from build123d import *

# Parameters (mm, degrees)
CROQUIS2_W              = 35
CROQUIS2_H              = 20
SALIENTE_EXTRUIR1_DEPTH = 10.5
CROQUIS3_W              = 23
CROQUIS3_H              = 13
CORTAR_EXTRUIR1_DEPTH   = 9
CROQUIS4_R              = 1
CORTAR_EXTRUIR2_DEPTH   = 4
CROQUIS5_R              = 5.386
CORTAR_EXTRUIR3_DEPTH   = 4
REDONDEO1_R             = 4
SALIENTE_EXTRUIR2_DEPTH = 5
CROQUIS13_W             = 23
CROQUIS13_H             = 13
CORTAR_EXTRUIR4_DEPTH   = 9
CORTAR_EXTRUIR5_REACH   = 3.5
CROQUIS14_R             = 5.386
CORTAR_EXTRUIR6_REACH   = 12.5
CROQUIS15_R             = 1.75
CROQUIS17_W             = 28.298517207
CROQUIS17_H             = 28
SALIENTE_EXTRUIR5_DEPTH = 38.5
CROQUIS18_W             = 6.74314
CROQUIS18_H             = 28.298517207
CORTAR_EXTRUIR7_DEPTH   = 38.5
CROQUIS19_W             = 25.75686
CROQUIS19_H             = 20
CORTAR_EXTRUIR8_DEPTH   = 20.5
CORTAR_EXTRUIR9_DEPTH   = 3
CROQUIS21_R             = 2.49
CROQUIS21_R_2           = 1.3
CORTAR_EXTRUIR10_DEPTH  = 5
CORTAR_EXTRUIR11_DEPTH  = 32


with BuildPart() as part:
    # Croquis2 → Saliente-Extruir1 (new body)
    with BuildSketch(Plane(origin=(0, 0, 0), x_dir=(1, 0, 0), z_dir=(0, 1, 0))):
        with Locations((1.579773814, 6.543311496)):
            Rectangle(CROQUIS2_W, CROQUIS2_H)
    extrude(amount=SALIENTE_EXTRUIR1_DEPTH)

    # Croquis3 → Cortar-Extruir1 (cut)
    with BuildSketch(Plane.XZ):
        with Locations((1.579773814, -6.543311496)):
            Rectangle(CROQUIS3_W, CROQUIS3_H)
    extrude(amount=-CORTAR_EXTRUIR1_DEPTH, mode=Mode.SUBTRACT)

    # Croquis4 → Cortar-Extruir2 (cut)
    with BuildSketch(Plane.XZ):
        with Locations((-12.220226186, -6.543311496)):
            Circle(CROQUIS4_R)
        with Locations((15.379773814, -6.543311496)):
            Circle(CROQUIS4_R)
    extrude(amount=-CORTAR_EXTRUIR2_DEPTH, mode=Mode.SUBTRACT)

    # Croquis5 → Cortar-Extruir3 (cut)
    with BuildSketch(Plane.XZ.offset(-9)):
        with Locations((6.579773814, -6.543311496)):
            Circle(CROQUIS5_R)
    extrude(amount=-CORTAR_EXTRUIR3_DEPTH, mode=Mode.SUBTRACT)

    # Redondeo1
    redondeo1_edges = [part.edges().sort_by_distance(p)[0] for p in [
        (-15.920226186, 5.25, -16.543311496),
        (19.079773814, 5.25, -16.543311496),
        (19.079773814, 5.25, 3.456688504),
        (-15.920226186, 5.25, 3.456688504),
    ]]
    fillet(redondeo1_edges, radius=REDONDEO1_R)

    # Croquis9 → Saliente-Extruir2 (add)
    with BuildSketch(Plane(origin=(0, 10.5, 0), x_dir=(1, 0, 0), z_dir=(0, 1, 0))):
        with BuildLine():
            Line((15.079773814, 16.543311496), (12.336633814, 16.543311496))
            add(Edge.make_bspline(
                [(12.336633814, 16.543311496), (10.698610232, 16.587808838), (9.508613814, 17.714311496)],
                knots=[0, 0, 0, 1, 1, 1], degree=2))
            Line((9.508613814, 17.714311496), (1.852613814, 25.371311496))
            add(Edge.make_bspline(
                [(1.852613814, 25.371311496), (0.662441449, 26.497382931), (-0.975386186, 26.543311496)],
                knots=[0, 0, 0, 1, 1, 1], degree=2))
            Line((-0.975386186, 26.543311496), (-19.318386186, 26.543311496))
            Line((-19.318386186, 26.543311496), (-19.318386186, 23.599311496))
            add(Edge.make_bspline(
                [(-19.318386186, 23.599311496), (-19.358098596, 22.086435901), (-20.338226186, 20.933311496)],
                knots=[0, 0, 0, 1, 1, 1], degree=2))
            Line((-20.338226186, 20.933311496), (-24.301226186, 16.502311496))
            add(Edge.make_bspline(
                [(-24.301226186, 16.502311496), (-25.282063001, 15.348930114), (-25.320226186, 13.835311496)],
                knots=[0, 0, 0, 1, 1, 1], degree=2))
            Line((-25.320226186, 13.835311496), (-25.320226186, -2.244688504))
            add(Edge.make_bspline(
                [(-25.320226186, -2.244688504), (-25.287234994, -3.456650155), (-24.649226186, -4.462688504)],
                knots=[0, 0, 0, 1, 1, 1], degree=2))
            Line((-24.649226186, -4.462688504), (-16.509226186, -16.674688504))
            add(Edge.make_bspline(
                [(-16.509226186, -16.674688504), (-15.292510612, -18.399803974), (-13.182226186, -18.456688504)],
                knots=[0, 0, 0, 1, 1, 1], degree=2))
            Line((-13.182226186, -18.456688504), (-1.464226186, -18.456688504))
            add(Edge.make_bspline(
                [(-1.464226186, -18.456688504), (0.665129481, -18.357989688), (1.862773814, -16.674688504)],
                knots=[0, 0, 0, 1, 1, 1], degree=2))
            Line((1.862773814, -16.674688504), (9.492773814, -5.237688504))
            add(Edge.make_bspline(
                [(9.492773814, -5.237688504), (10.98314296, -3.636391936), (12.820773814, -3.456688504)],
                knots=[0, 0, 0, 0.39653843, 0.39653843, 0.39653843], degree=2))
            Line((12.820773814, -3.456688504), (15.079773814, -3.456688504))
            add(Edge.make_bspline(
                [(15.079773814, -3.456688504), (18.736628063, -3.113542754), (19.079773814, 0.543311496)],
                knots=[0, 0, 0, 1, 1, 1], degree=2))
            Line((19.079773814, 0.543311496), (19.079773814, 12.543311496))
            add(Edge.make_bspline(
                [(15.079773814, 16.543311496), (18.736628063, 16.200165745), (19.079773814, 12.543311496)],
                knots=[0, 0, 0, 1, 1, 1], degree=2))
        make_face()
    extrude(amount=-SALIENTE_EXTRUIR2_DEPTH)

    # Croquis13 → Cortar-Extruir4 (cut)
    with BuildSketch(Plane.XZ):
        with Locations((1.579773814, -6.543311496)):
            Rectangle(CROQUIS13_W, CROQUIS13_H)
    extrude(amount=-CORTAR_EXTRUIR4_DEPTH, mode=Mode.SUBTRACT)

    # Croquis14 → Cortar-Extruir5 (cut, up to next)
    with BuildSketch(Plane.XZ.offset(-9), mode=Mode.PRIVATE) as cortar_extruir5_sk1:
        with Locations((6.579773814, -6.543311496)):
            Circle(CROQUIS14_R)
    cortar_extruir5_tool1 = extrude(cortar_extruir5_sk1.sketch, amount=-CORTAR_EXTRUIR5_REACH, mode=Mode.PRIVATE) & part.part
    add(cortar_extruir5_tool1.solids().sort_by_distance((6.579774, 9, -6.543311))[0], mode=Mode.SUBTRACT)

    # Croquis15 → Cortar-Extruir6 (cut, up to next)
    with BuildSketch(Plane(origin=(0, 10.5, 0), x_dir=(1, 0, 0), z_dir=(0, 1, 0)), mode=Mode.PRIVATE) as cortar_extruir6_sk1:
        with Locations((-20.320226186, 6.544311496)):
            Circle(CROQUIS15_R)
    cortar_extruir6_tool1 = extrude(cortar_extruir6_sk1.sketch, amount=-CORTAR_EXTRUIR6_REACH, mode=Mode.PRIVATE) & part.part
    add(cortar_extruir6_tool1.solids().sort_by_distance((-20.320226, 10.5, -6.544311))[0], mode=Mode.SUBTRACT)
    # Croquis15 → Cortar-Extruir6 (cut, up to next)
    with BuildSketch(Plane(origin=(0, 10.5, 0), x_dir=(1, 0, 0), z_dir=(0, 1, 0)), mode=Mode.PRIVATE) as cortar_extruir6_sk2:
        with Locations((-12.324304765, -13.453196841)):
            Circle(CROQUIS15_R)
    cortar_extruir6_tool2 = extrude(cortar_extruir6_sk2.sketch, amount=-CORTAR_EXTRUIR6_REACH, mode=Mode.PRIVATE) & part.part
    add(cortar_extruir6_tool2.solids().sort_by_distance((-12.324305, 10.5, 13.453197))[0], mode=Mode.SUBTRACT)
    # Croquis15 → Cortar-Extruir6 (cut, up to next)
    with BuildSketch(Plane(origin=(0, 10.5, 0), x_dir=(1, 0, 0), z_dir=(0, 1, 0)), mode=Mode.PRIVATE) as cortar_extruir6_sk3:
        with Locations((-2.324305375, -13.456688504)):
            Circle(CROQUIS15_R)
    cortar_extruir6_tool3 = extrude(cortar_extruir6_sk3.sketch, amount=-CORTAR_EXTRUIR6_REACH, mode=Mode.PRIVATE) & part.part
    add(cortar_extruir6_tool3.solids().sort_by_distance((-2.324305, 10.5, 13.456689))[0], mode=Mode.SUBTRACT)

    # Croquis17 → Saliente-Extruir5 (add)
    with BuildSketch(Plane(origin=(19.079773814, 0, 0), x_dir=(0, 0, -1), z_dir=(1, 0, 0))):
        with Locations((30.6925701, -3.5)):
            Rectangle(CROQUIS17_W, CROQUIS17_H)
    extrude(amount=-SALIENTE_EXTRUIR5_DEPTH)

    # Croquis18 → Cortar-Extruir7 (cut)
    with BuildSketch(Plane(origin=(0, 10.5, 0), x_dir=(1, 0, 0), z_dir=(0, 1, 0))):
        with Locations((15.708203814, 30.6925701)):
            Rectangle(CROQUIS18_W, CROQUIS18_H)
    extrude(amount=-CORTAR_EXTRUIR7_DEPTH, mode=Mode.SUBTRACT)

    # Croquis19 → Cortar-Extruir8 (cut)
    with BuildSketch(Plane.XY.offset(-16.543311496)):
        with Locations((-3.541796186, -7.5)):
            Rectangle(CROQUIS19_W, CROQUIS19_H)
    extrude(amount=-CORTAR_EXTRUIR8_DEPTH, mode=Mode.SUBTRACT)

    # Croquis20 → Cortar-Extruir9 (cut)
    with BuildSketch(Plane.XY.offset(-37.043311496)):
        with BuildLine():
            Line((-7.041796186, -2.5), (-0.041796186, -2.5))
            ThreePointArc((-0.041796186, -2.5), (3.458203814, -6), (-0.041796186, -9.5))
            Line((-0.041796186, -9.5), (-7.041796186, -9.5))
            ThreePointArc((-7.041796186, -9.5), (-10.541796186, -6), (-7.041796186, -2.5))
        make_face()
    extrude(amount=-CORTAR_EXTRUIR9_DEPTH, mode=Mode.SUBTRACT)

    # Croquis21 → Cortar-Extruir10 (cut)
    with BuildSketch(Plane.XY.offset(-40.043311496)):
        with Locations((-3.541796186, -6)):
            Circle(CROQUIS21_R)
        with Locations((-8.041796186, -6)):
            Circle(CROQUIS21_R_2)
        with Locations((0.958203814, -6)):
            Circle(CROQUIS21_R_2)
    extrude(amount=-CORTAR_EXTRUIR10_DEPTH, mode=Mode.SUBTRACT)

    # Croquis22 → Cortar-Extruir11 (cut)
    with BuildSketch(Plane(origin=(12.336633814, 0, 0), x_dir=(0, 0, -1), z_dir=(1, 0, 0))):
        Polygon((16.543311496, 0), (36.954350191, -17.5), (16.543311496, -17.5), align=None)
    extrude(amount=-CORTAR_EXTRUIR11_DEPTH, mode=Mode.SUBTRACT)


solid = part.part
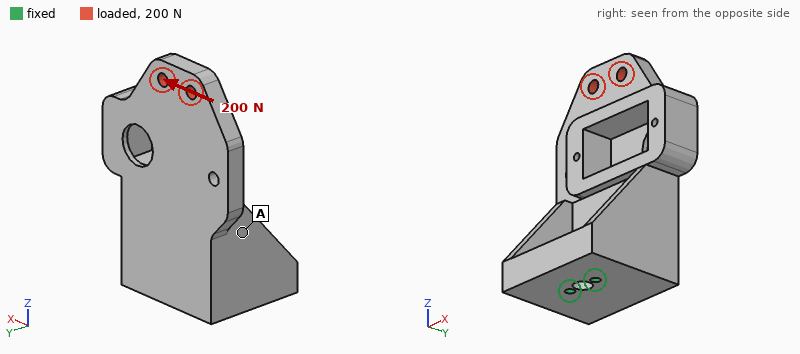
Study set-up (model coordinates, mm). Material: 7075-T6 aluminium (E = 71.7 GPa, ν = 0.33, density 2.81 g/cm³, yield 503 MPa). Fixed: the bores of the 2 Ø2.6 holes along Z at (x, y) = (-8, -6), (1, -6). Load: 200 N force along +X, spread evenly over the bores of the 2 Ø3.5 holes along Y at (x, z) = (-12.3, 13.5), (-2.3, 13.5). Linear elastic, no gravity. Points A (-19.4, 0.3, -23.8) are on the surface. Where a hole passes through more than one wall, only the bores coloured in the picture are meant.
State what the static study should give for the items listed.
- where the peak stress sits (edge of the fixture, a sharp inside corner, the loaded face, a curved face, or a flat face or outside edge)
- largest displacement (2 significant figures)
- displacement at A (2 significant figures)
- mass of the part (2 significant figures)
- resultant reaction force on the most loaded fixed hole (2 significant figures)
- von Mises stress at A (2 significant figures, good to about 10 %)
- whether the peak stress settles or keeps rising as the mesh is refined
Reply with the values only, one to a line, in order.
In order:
edge of the fixture
71 µm
25 µm
57 g
830 N
4.9 MPa
keeps rising
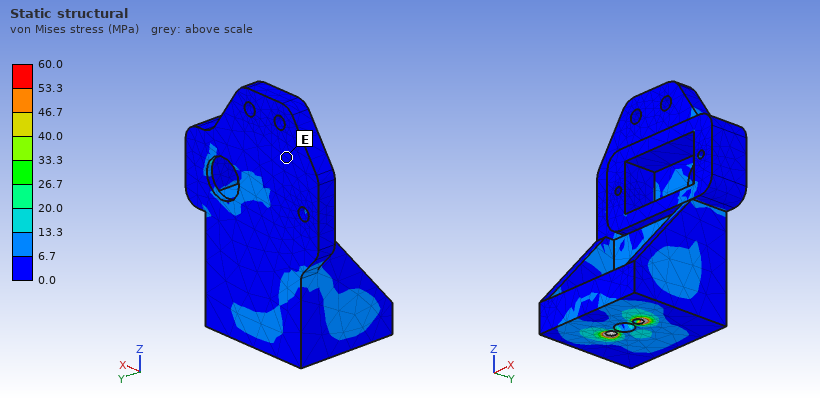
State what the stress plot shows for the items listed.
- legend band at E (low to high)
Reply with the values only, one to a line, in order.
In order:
0.0 to 6.7 MPa
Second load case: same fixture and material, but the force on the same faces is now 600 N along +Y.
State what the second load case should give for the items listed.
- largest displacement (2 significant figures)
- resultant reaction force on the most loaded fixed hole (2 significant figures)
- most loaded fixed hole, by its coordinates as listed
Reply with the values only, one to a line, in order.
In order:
0.66 mm
510 N
(-8, -6)
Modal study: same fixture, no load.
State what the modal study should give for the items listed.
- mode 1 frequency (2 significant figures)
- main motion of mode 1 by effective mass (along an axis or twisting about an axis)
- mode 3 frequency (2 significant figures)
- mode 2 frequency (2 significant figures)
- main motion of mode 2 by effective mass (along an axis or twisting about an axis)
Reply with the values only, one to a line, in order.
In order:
1600 Hz
along Y
5300 Hz
2400 Hz
along X
